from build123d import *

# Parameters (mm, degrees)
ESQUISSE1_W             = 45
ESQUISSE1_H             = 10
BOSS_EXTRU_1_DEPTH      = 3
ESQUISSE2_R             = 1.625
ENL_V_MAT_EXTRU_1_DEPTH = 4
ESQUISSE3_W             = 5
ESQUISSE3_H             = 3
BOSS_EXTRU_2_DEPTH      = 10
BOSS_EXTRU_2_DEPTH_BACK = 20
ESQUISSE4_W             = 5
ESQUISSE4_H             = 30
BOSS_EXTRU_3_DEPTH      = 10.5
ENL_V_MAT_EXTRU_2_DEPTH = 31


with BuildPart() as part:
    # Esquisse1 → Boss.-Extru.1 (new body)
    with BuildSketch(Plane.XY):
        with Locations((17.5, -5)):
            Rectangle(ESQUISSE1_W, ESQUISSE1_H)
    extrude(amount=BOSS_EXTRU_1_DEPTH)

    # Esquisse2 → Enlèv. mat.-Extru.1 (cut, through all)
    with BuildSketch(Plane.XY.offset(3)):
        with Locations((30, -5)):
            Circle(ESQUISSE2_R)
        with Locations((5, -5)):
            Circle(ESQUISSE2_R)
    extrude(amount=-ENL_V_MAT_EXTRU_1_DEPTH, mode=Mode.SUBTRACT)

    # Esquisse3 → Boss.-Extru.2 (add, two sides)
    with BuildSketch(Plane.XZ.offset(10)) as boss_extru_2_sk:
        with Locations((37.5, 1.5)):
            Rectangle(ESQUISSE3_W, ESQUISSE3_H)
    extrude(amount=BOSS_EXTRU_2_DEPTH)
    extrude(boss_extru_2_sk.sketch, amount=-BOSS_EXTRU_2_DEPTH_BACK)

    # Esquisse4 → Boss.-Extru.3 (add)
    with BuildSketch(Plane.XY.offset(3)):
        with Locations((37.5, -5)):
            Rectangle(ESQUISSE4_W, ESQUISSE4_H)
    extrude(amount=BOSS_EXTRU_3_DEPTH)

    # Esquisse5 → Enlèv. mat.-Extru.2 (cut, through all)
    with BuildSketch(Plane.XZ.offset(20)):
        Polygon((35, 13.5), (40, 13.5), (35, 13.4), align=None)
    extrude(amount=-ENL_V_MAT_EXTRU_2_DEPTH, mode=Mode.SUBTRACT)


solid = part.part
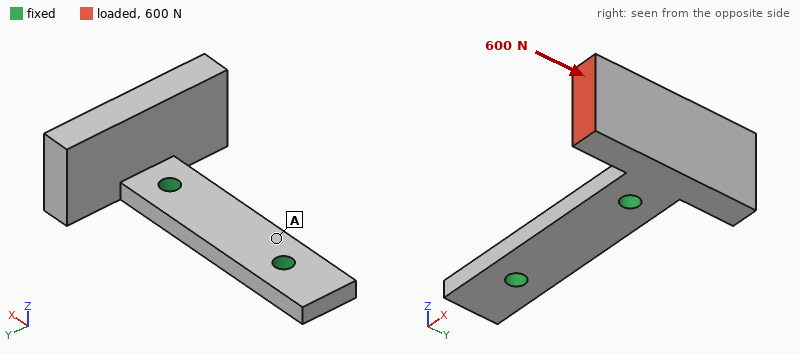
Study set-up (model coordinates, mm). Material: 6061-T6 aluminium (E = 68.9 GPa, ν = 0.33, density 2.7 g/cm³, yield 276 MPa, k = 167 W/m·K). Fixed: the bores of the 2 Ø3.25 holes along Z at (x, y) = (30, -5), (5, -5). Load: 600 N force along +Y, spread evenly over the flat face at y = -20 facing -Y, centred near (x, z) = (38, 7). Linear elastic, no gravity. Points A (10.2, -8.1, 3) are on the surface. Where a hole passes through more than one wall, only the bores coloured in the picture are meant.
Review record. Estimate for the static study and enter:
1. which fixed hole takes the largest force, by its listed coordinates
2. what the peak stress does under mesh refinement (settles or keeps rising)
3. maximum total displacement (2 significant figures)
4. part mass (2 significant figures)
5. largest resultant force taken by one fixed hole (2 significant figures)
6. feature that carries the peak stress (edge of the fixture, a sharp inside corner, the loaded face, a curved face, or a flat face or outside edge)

(30, -5)
keeps rising
0.13 mm
8.6 g
680 N
edge of the fixture
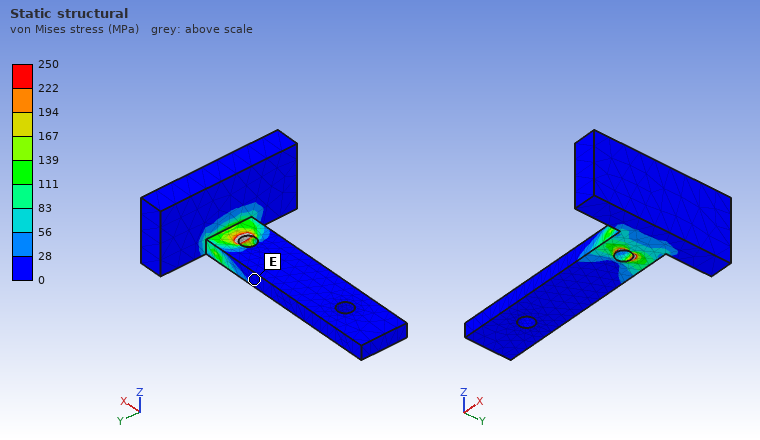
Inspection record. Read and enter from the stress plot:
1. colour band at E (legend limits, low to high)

0 to 28 MPa
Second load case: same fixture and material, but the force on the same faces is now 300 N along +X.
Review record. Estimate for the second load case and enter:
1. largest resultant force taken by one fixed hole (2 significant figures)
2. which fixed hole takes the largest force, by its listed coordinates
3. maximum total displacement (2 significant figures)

300 N
(30, -5)
0.16 mm
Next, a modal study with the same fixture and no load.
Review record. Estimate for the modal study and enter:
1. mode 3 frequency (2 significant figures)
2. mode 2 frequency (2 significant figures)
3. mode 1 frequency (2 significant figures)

7800 Hz
4600 Hz
4400 Hz
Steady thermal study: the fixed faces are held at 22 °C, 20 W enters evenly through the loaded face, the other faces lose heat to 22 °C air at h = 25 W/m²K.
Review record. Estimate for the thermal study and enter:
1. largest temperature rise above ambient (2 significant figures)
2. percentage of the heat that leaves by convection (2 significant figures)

49 K
4.4 %
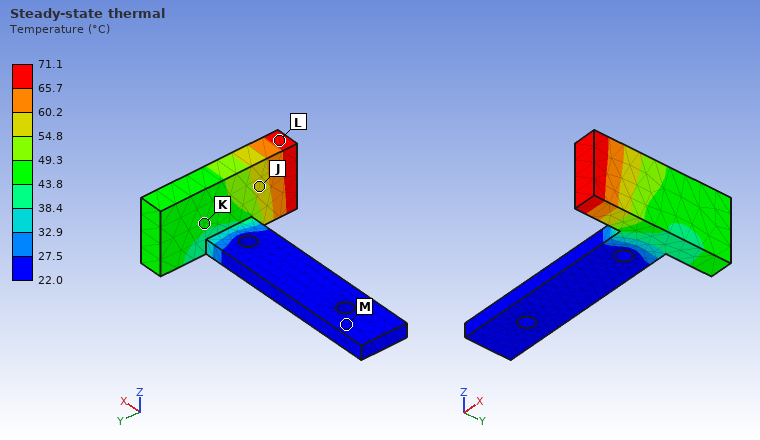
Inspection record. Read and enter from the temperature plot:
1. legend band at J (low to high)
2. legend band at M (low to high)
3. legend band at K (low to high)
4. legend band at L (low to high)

54.8 to 60.2 °C
22.0 to 27.5 °C
43.8 to 49.3 °C
65.7 to 71.1 °C
